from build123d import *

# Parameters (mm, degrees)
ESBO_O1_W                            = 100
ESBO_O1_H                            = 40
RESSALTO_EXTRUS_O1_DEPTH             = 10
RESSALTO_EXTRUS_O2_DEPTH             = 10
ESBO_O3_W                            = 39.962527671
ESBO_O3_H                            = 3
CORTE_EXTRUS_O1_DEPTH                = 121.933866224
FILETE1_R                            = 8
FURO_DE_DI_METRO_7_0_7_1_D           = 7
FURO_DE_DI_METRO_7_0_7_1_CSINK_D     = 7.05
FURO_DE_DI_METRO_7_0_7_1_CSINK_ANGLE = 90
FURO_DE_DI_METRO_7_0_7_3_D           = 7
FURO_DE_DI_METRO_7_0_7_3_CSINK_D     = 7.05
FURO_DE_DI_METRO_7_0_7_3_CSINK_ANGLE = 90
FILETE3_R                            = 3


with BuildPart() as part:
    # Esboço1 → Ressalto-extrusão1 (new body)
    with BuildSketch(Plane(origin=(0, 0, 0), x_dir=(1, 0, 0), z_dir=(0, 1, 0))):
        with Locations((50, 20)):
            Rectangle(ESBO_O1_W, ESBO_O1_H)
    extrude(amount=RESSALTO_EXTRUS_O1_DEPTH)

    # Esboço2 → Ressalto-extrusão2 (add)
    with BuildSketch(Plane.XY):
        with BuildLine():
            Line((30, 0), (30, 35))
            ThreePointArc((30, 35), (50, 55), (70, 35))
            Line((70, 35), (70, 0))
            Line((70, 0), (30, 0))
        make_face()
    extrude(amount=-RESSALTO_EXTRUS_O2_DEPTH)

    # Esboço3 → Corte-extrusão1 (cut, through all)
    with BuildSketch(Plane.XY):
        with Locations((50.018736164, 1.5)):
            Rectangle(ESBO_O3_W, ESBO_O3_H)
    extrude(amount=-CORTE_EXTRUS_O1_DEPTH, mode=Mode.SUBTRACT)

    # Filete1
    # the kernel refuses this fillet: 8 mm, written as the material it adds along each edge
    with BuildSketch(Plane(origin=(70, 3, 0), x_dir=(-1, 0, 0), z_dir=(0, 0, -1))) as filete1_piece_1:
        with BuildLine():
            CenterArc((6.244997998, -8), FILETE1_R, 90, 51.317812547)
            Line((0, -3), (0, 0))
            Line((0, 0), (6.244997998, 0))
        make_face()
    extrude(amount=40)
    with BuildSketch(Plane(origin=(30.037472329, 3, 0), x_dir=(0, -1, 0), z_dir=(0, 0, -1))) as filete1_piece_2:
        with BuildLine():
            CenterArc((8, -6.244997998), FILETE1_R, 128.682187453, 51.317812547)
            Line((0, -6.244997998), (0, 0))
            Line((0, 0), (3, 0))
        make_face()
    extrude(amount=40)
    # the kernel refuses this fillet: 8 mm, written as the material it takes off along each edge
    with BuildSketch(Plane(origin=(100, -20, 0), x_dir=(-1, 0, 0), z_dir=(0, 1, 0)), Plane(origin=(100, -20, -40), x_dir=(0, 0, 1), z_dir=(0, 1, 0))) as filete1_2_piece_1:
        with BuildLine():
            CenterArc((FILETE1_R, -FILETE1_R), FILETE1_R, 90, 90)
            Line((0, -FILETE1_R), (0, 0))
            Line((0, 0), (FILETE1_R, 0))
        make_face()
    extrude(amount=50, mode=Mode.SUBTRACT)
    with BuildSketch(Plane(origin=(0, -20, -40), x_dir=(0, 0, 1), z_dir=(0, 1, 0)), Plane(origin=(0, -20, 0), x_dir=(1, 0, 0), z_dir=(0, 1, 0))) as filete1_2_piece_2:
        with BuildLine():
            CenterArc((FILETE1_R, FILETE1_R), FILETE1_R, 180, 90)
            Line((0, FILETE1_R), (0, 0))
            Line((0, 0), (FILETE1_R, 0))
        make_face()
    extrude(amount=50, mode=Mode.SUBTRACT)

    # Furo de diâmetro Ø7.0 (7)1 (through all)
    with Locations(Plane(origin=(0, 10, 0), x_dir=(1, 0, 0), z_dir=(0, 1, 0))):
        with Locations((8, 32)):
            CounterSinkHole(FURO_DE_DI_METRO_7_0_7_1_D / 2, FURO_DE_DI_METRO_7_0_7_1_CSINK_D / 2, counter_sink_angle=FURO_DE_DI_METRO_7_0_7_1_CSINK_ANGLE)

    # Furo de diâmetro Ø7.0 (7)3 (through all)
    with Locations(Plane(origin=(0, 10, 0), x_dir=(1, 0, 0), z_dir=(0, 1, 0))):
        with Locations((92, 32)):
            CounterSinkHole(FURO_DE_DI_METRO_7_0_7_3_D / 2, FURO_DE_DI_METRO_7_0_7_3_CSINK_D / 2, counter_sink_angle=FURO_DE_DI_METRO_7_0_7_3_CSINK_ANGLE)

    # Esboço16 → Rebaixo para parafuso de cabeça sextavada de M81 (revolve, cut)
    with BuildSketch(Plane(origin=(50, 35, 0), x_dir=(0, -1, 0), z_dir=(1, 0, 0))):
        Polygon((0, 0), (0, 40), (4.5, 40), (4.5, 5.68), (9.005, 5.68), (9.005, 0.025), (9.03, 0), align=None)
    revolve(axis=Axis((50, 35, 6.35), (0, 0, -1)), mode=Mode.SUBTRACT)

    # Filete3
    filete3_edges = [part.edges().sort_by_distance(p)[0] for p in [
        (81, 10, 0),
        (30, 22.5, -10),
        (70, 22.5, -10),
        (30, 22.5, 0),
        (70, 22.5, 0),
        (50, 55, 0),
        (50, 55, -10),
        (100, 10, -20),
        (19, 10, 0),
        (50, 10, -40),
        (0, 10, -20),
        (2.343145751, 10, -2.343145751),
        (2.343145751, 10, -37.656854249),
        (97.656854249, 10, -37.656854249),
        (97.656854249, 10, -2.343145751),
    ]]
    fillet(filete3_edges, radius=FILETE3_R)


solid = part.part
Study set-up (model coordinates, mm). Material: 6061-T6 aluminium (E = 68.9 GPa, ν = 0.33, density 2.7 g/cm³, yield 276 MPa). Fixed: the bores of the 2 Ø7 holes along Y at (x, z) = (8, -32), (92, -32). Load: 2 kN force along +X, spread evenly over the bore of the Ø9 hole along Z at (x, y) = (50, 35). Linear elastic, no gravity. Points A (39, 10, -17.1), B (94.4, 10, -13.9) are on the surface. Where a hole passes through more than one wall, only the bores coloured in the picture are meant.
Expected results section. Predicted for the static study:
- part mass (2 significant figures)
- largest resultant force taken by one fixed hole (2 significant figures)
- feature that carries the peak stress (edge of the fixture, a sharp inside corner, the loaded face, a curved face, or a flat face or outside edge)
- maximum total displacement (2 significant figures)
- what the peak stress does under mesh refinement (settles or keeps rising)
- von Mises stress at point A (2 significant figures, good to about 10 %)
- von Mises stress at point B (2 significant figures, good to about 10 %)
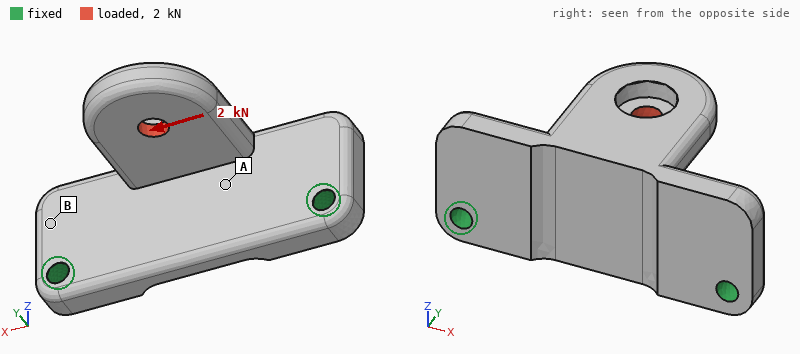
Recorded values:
130 g
1.4 kN
edge of the fixture
0.11 mm
keeps rising
31 MPa
10 MPa
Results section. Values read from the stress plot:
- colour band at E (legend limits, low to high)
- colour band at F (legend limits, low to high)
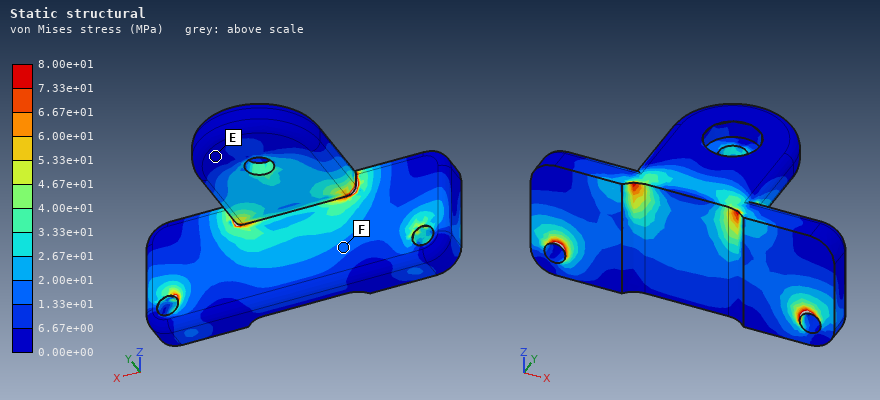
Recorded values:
0.00e+00 to 6.67e+00 MPa
1.33e+01 to 2.00e+01 MPa
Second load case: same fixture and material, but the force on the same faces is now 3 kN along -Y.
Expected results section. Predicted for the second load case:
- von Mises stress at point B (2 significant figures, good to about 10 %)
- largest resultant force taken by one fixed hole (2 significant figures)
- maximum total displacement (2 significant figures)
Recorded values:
32 MPa
1.6 kN
0.20 mm
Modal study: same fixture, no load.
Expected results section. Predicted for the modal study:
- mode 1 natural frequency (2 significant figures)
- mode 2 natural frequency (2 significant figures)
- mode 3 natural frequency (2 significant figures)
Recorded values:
2000 Hz
4000 Hz
4200 Hz
